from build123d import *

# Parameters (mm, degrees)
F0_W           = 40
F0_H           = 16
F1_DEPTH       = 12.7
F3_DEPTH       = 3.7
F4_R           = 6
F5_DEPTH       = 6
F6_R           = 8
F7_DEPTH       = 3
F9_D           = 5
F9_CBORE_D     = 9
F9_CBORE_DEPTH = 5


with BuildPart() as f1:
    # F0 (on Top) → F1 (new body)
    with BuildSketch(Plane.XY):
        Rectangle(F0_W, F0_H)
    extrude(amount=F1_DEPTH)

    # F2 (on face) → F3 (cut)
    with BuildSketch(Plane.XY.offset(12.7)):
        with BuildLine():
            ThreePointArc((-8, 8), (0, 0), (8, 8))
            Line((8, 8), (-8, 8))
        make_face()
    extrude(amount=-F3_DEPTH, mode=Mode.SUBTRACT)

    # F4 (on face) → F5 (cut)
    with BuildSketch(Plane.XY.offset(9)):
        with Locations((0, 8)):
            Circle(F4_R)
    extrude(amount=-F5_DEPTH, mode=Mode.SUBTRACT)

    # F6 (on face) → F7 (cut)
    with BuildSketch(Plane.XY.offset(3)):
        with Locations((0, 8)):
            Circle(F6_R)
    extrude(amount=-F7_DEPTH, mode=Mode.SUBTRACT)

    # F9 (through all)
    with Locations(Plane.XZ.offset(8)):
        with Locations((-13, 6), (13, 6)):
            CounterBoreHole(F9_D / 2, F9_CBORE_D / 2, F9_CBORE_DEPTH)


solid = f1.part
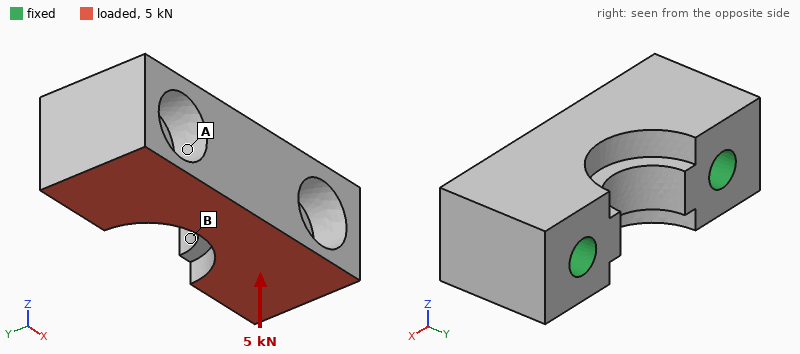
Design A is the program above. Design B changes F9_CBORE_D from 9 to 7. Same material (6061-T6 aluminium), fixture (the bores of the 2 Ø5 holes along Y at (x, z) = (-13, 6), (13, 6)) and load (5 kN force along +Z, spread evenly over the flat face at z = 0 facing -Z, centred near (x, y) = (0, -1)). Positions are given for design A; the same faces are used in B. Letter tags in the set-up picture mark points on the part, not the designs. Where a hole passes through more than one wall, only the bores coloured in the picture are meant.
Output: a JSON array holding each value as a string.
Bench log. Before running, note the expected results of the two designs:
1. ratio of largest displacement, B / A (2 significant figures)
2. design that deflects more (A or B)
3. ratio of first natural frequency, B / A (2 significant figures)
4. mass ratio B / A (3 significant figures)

["0.75", "A", "1.1", "1.04"]
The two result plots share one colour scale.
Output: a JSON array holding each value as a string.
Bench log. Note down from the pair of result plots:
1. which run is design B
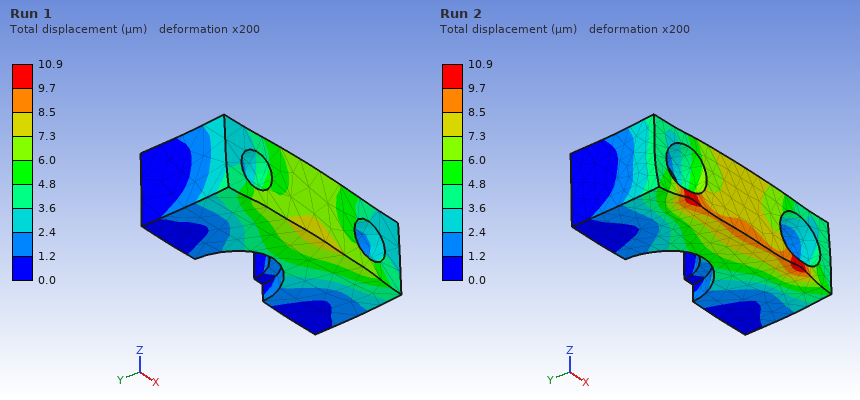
["Run 1"]
